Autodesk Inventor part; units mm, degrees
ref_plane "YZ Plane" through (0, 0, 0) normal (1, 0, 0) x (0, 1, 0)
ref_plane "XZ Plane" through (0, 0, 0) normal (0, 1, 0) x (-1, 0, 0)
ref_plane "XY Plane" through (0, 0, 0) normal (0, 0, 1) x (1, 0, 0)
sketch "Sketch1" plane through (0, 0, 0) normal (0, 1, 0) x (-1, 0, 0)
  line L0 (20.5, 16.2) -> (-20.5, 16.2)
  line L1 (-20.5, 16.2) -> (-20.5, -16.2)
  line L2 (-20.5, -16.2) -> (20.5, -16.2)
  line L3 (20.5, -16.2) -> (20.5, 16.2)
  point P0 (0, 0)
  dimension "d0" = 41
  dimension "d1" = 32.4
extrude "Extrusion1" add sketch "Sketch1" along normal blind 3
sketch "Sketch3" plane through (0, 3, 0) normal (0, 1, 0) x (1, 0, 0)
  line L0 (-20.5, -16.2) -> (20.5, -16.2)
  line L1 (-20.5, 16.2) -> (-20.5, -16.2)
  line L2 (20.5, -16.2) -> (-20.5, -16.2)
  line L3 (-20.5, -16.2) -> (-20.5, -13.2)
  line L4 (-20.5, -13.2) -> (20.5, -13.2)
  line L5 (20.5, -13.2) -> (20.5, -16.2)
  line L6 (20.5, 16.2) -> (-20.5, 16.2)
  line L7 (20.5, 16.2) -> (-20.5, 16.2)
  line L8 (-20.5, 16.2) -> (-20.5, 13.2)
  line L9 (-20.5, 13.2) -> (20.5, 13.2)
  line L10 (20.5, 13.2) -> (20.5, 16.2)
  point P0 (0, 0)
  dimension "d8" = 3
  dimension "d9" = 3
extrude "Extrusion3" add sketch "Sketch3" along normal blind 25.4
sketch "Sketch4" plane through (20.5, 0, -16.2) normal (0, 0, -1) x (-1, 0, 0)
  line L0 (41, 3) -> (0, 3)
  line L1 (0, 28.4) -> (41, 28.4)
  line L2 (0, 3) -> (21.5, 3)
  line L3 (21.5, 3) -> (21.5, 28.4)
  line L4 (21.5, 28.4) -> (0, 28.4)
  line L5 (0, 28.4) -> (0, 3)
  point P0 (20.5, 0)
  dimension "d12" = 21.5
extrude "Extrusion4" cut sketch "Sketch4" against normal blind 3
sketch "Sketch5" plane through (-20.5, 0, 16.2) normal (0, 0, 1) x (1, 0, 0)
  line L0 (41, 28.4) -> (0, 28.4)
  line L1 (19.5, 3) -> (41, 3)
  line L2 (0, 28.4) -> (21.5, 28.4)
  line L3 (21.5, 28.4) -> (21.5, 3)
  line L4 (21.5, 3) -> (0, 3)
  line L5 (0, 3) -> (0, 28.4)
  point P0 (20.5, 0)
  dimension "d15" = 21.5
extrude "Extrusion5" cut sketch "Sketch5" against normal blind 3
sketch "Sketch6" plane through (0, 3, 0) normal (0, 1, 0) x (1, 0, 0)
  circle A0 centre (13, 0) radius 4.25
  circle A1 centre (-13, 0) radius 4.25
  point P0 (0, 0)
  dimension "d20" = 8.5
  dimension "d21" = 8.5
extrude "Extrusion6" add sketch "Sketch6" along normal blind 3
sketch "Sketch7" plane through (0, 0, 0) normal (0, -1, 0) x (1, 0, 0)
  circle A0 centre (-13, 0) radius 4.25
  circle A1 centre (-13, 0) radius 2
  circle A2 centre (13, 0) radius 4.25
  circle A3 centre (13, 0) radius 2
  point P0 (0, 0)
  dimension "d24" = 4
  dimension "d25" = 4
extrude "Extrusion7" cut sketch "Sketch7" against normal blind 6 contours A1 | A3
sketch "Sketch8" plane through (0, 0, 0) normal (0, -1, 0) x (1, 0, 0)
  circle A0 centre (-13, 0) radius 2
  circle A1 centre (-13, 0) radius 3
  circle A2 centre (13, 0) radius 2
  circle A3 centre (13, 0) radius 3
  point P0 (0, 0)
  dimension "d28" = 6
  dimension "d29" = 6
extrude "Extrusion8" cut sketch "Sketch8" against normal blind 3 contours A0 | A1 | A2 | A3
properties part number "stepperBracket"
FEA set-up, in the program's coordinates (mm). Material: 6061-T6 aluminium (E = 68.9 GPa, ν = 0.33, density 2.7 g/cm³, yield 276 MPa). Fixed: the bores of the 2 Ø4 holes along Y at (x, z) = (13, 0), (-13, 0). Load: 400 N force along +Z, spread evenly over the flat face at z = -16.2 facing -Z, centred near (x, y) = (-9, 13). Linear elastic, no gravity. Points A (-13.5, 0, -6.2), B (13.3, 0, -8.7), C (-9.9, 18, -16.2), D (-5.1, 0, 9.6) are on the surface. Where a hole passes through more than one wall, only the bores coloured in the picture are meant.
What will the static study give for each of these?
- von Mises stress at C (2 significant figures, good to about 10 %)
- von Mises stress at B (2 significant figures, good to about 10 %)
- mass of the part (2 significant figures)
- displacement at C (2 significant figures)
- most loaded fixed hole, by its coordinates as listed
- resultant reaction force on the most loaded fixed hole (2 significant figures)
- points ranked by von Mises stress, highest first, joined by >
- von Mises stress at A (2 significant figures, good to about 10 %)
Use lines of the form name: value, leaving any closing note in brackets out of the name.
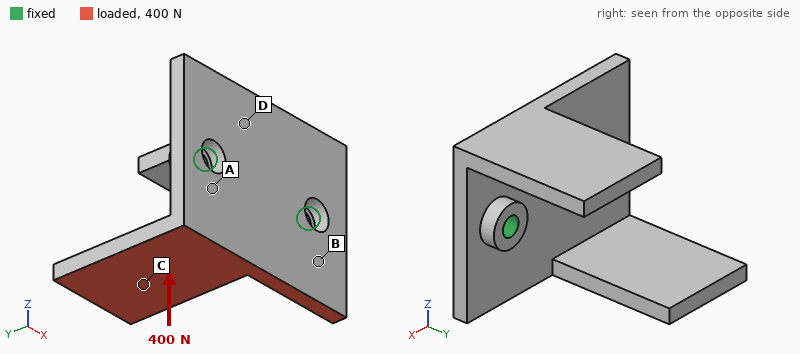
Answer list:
von Mises stress at C: 24 MPa
von Mises stress at B: 37 MPa
mass of the part: 19 g
displacement at C: 0.38 mm
most loaded fixed hole, by its coordinates as listed: (-13, 0)
resultant reaction force on the most loaded fixed hole: 340 N
points ranked by von Mises stress, highest first, joined by >: A > B > C > D
von Mises stress at A: 91 MPa
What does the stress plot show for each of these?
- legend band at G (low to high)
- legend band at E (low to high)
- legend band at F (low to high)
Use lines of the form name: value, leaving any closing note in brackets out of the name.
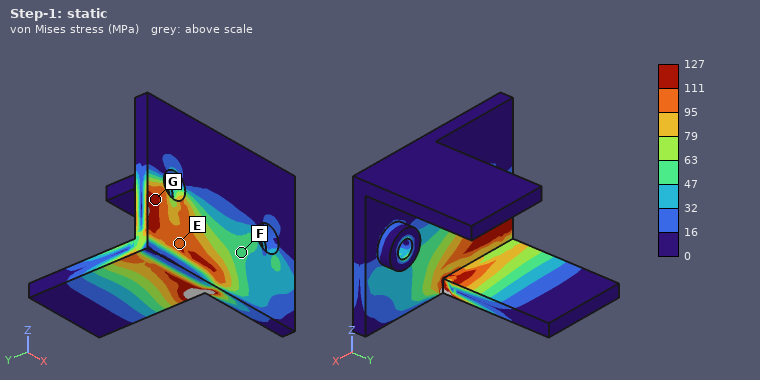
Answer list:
legend band at G: 111 to 127 MPa
legend band at E: 95 to 111 MPa
legend band at F: 47 to 63 MPa
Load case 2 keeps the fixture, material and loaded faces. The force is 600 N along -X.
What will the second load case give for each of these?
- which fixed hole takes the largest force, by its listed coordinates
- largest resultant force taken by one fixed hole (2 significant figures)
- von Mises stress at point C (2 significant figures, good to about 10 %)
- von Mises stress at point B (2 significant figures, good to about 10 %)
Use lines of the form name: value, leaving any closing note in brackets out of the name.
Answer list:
which fixed hole takes the largest force, by its listed coordinates: (-13, 0)
largest resultant force taken by one fixed hole: 690 N
von Mises stress at point C: 16 MPa
von Mises stress at point B: 27 MPa
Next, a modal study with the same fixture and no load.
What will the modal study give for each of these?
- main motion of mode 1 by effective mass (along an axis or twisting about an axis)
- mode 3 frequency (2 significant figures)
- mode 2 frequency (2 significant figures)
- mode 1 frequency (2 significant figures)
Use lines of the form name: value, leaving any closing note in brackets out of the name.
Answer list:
main motion of mode 1 by effective mass: along Z
mode 3 frequency: 3700 Hz
mode 2 frequency: 2100 Hz
mode 1 frequency: 2000 Hz
